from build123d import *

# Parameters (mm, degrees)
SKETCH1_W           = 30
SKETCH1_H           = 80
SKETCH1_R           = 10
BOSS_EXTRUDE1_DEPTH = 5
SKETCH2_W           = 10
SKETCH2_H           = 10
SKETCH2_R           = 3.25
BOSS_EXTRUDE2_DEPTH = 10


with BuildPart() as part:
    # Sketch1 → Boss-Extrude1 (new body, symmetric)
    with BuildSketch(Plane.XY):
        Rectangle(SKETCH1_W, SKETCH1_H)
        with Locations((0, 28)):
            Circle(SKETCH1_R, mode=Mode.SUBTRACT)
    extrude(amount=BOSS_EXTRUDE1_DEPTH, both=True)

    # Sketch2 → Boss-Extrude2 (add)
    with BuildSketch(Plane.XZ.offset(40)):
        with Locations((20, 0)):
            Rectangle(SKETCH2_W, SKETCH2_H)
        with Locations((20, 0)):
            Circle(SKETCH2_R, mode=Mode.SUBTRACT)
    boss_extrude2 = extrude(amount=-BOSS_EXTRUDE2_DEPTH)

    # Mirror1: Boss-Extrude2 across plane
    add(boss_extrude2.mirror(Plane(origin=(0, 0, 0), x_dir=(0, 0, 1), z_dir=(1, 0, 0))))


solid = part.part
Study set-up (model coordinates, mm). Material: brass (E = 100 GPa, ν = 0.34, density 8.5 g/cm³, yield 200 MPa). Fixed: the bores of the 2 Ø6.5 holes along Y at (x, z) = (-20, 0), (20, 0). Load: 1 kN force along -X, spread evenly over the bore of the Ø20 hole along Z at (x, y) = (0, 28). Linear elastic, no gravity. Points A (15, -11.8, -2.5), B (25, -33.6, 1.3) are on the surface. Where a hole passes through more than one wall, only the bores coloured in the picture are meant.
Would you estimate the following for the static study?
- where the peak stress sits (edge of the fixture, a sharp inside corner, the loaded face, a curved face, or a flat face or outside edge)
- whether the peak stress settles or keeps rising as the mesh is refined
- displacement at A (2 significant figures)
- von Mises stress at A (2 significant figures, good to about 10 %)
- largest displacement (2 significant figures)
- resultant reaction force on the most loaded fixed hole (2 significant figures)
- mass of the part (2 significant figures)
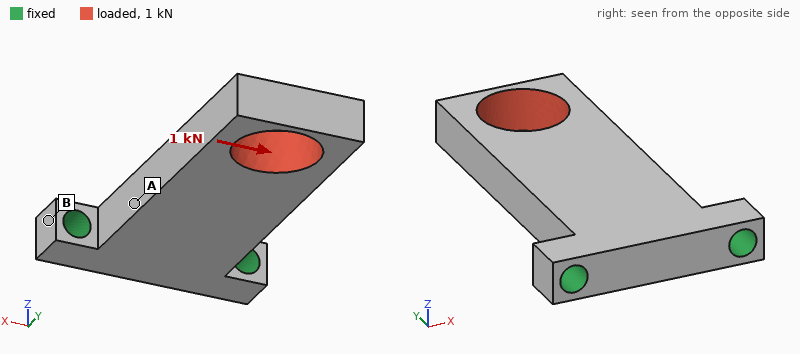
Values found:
edge of the fixture
keeps rising
15 µm
26 MPa
80 µm
2.0 kN
190 g
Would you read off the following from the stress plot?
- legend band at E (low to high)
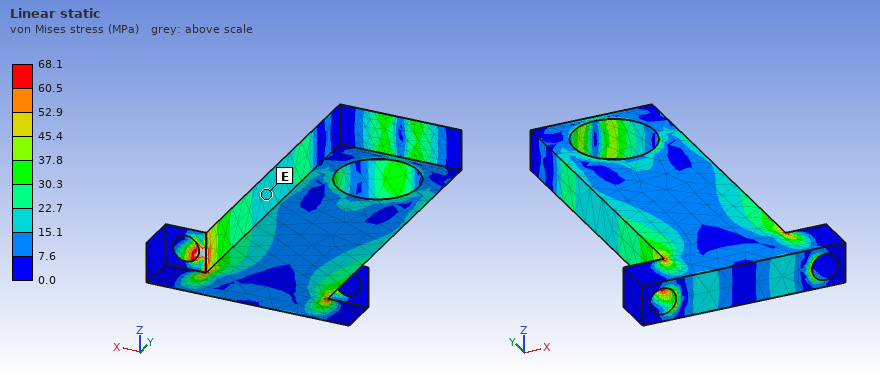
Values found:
15.1 to 22.7 MPa
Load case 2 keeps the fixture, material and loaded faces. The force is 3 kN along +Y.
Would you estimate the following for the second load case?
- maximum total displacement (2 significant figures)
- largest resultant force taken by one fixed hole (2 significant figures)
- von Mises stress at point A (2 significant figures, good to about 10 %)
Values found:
24 µm
1.6 kN
10.0 MPa
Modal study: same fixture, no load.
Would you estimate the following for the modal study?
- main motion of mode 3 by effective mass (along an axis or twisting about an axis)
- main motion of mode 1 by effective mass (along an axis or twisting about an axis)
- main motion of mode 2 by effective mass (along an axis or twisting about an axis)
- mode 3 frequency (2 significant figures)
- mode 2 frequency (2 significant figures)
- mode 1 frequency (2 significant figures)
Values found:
twisting about Y
along Z
along X
4100 Hz
2900 Hz
930 Hz
